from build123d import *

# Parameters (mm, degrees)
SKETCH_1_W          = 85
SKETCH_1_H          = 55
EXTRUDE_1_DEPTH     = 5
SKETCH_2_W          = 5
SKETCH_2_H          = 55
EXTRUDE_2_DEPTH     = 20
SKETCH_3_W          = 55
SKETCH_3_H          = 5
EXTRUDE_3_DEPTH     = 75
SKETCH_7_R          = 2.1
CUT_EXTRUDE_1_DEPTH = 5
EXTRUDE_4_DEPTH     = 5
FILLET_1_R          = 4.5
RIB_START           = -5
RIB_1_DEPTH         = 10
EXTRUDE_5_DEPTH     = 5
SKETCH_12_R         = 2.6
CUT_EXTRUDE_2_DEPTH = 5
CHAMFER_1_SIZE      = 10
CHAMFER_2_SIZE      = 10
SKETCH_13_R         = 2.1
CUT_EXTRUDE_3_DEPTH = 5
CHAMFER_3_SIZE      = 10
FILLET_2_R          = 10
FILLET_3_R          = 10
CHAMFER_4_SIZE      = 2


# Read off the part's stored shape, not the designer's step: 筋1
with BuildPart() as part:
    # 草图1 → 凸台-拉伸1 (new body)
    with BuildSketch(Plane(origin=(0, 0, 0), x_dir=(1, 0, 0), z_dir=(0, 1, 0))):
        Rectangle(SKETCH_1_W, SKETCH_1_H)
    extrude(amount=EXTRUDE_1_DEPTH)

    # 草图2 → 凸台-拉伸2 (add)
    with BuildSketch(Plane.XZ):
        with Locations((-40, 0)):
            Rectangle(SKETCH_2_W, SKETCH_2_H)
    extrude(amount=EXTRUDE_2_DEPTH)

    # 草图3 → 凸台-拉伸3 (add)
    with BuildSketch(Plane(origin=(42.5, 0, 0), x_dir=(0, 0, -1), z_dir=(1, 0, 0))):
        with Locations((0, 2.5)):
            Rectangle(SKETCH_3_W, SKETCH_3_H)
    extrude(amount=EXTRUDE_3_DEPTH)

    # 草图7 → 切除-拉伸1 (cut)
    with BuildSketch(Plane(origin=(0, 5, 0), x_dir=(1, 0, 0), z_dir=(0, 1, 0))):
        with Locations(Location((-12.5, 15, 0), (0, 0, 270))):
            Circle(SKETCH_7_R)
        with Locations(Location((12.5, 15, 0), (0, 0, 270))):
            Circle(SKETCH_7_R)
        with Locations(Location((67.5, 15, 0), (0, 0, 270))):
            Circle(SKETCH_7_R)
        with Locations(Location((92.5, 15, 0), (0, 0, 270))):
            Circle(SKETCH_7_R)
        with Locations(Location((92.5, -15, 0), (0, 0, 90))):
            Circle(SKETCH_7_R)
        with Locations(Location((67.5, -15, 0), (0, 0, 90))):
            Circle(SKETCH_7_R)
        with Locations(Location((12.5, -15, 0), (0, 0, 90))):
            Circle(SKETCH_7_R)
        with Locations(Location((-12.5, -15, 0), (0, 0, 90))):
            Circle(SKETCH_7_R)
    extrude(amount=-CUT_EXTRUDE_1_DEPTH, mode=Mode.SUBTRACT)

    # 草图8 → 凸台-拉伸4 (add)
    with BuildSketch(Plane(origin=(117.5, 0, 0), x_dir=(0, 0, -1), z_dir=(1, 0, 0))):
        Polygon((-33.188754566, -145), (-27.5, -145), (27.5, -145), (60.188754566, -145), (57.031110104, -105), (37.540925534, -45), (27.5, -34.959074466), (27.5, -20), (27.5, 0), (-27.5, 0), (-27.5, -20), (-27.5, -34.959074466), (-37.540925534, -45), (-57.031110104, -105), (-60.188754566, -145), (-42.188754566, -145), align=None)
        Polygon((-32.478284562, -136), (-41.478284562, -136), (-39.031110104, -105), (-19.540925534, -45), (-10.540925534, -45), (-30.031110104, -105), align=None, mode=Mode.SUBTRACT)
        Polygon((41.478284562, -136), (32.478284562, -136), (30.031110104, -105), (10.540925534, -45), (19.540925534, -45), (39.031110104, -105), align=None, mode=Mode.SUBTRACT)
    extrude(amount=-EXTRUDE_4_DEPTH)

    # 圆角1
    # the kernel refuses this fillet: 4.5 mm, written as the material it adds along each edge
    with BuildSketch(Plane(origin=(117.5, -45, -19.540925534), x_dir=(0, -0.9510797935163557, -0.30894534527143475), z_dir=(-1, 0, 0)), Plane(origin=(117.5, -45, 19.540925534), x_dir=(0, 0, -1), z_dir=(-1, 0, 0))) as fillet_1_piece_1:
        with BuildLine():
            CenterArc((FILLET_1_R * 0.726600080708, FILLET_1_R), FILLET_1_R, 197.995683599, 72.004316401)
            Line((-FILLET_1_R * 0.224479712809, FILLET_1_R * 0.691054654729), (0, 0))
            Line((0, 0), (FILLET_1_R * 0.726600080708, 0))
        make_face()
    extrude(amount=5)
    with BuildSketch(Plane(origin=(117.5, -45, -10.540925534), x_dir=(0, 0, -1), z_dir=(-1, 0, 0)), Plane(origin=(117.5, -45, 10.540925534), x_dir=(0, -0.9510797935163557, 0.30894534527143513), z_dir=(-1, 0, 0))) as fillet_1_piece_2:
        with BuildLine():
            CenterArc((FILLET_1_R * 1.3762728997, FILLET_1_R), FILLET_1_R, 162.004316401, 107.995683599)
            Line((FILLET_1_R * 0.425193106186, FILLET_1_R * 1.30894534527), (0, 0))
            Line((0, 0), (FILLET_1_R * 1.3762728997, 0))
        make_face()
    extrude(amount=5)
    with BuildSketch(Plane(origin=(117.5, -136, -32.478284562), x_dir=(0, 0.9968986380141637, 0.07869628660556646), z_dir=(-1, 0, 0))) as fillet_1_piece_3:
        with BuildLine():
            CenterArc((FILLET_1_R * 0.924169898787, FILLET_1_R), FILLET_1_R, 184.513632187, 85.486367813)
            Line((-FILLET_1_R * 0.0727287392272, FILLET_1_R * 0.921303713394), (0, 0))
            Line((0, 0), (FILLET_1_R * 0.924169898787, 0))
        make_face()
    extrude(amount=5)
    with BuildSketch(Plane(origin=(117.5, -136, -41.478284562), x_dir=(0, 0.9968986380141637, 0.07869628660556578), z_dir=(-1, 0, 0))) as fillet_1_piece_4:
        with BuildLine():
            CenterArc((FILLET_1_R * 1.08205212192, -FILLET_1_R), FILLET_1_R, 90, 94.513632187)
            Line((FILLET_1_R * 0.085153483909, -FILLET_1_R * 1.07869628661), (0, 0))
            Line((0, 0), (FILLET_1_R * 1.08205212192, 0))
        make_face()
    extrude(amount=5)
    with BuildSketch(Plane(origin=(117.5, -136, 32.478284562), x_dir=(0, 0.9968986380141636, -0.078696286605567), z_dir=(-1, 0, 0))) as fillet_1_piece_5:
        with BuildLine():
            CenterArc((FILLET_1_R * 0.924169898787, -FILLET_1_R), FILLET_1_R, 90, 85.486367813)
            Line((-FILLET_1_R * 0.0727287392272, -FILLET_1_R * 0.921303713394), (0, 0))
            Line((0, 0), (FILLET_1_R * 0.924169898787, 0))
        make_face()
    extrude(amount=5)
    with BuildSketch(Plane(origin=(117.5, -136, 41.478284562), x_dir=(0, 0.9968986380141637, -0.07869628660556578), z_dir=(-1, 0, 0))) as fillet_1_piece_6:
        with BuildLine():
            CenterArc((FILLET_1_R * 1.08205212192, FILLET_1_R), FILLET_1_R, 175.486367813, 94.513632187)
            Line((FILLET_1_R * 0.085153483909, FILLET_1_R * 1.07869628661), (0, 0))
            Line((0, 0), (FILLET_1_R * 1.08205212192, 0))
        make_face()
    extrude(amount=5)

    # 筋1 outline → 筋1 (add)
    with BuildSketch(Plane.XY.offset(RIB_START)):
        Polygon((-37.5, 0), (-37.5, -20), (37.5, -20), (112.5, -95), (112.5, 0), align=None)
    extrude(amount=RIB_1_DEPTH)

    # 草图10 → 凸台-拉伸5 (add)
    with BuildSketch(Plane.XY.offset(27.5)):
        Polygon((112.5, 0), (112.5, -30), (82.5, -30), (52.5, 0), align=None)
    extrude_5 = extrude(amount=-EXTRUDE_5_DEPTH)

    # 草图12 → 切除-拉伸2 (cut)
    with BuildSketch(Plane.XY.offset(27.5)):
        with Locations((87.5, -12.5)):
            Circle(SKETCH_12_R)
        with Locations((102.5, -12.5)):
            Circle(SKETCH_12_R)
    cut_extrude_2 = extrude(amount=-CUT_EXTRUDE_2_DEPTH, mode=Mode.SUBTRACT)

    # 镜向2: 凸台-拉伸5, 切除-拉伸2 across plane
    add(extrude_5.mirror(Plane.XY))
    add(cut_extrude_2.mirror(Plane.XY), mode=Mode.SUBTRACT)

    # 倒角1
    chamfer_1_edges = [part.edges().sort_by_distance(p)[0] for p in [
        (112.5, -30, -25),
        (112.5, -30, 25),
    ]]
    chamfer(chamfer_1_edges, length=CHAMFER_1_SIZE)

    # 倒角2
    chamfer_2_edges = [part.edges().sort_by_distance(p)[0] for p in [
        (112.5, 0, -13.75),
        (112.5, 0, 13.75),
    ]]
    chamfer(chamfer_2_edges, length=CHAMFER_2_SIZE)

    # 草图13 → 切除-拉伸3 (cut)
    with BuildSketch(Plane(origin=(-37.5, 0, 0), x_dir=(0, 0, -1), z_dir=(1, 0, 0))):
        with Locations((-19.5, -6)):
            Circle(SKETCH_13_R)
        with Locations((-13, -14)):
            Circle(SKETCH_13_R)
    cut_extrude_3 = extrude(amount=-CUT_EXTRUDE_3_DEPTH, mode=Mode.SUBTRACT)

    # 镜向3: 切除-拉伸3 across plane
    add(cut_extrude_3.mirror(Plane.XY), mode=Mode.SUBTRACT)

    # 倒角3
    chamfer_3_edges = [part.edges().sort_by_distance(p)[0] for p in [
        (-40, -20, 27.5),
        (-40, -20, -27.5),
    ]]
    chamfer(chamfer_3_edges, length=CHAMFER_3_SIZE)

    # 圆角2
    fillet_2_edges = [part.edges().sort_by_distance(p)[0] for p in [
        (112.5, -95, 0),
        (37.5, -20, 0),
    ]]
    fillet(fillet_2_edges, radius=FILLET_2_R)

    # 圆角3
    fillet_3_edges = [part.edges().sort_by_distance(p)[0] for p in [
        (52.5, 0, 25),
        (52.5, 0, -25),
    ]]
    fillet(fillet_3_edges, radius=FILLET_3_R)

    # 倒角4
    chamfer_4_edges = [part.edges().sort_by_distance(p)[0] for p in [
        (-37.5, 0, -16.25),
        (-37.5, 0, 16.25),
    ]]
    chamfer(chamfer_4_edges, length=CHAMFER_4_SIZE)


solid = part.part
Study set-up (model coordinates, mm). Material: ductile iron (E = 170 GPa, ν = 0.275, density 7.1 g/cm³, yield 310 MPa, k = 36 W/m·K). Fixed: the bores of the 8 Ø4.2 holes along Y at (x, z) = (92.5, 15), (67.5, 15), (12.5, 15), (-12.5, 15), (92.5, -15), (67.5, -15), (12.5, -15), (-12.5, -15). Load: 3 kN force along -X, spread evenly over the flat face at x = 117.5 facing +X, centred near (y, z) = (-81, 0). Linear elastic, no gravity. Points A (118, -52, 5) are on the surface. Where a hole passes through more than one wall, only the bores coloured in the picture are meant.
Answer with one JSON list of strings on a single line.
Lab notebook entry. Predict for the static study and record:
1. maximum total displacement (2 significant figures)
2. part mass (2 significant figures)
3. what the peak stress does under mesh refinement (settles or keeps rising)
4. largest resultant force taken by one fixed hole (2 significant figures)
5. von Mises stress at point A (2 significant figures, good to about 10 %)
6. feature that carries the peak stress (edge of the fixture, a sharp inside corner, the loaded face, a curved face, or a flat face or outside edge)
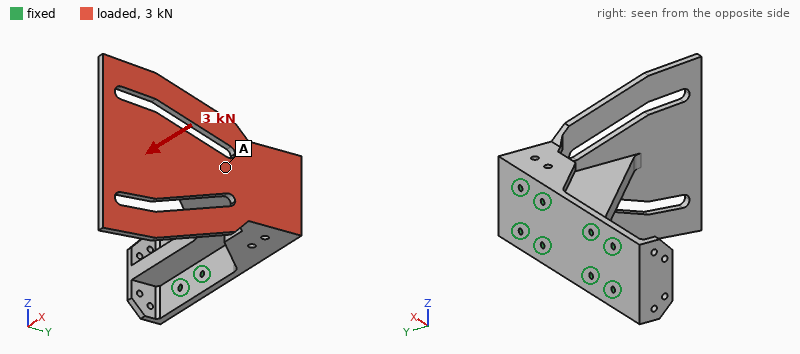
["0.65 mm", "1.3 kg", "keeps rising", "2.2 kN", "21 MPa", "a sharp inside corner"]
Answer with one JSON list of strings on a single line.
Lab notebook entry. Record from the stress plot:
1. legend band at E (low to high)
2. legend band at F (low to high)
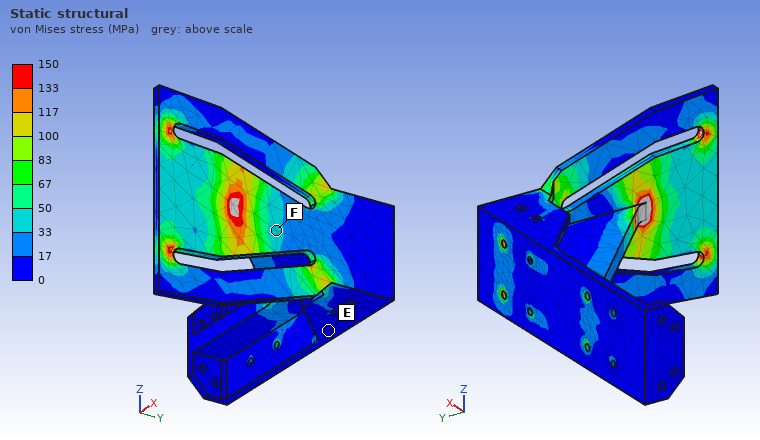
["0 to 17 MPa", "33 to 50 MPa"]
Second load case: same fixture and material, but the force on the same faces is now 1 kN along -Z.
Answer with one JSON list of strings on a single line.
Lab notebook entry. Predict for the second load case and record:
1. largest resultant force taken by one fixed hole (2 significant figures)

["2.2 kN"]
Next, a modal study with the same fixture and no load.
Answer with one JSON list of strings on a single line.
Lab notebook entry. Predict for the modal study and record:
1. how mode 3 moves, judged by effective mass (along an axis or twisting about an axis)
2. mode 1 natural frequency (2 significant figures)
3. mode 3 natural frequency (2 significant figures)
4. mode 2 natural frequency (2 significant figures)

["along Z", "690 Hz", "740 Hz", "690 Hz"]
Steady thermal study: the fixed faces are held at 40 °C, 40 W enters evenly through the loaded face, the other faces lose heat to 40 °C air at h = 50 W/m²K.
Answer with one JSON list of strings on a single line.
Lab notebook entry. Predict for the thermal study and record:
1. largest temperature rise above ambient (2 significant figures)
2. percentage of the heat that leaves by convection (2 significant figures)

["41 K", "78 %"]
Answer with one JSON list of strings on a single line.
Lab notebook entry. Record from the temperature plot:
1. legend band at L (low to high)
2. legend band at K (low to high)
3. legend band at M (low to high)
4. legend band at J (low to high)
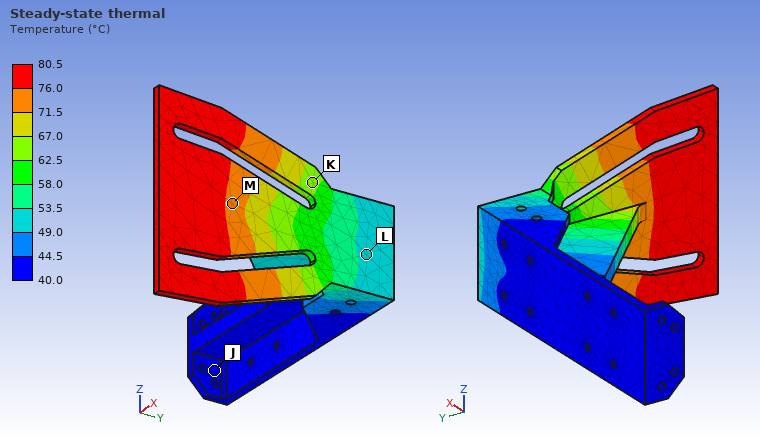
["49.0 to 53.5 °C", "62.5 to 67.0 °C", "71.5 to 76.0 °C", "40.0 to 44.5 °C"]
